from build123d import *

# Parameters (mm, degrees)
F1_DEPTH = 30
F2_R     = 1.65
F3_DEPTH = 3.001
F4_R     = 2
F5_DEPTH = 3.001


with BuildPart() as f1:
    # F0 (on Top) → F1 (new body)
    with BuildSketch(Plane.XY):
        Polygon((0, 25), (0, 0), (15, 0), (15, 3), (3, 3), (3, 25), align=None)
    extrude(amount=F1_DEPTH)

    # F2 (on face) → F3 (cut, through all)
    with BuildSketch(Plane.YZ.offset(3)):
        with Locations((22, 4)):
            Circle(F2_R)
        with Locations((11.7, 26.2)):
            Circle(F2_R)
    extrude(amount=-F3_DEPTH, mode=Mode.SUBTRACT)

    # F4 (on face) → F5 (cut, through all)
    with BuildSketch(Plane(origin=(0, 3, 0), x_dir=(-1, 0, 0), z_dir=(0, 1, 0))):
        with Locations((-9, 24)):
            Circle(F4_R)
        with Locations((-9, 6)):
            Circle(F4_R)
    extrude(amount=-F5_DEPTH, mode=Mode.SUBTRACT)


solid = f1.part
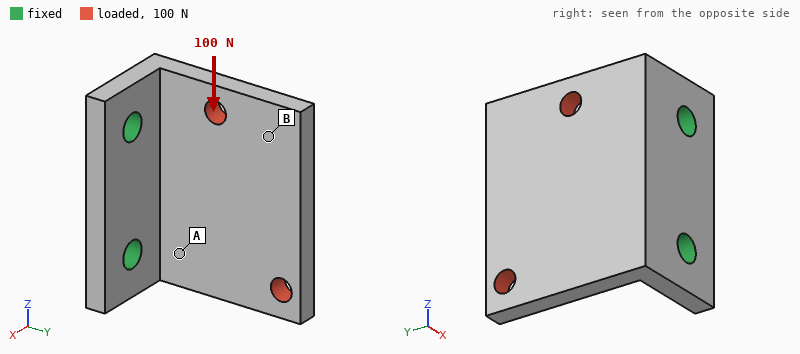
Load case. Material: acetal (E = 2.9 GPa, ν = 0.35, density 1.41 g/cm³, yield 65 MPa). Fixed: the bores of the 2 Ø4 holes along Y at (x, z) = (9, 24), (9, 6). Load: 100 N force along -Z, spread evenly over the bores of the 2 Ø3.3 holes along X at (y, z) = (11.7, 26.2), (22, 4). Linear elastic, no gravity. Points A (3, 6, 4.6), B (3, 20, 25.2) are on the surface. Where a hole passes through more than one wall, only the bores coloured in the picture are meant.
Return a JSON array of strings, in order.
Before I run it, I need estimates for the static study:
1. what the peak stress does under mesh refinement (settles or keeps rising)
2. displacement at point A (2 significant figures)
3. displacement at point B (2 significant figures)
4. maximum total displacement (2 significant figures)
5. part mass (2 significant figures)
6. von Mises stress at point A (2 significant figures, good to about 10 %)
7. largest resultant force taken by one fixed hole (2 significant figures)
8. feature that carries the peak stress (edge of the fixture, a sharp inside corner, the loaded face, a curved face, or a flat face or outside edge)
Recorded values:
["keeps rising", "0.081 mm", "0.19 mm", "0.26 mm", "4.5 g", "6.7 MPa", "96 N", "edge of the fixture"]
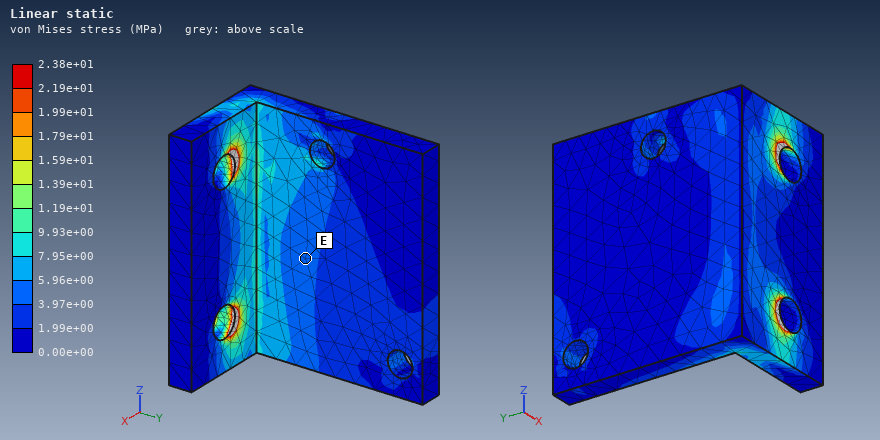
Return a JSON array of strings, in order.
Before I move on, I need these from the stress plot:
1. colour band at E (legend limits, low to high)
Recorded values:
["3.97e+00 to 5.96e+00 MPa"]
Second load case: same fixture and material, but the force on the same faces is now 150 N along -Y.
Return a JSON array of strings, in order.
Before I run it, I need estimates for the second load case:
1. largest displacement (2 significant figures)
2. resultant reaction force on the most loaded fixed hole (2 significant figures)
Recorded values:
["0.44 mm", "76 N"]
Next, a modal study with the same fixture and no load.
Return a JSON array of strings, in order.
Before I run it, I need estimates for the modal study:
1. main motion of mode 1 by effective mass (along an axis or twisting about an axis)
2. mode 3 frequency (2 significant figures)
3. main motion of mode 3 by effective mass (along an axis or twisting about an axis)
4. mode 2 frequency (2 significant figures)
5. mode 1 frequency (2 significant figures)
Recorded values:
["along X", "3000 Hz", "along Z", "2000 Hz", "920 Hz"]
